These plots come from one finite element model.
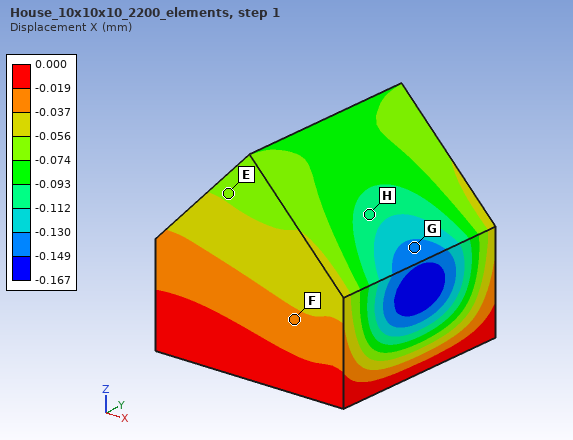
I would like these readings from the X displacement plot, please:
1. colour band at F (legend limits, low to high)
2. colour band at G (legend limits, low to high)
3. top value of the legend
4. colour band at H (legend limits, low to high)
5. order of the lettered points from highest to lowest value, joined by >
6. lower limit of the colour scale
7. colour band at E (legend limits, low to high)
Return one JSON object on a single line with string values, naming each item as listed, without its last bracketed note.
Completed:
{"colour band at F": "-0.037 to -0.019 mm", "colour band at G": "-0.149 to -0.130 mm", "top value of the legend": "0.000 mm", "colour band at H": "-0.112 to -0.093 mm", "order of the lettered points from highest to lowest value, joined by >": "F > E > H > G", "lower limit of the colour scale": "-0.167 mm", "colour band at E": "-0.074 to -0.056 mm"}
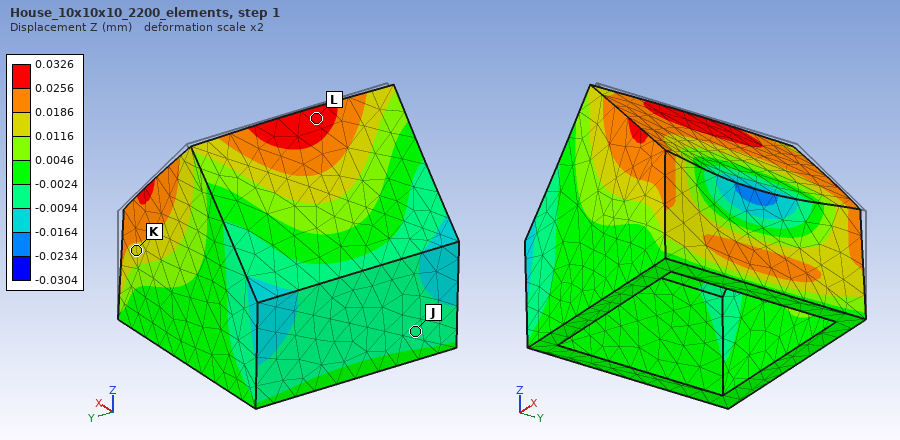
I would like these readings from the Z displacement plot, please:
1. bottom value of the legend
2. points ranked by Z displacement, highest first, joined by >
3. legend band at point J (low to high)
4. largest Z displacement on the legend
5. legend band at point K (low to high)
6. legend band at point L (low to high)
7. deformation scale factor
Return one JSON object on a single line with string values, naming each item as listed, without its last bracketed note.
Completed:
{"bottom value of the legend": "-0.0304 mm", "points ranked by Z displacement, highest first, joined by >": "L > K > J", "legend band at point J": "-0.0094 to -0.0024 mm", "largest Z displacement on the legend": "0.0326 mm", "legend band at point K": "0.0116 to 0.0186 mm", "legend band at point L": "0.0256 to 0.0326 mm", "deformation scale factor": "2"}
